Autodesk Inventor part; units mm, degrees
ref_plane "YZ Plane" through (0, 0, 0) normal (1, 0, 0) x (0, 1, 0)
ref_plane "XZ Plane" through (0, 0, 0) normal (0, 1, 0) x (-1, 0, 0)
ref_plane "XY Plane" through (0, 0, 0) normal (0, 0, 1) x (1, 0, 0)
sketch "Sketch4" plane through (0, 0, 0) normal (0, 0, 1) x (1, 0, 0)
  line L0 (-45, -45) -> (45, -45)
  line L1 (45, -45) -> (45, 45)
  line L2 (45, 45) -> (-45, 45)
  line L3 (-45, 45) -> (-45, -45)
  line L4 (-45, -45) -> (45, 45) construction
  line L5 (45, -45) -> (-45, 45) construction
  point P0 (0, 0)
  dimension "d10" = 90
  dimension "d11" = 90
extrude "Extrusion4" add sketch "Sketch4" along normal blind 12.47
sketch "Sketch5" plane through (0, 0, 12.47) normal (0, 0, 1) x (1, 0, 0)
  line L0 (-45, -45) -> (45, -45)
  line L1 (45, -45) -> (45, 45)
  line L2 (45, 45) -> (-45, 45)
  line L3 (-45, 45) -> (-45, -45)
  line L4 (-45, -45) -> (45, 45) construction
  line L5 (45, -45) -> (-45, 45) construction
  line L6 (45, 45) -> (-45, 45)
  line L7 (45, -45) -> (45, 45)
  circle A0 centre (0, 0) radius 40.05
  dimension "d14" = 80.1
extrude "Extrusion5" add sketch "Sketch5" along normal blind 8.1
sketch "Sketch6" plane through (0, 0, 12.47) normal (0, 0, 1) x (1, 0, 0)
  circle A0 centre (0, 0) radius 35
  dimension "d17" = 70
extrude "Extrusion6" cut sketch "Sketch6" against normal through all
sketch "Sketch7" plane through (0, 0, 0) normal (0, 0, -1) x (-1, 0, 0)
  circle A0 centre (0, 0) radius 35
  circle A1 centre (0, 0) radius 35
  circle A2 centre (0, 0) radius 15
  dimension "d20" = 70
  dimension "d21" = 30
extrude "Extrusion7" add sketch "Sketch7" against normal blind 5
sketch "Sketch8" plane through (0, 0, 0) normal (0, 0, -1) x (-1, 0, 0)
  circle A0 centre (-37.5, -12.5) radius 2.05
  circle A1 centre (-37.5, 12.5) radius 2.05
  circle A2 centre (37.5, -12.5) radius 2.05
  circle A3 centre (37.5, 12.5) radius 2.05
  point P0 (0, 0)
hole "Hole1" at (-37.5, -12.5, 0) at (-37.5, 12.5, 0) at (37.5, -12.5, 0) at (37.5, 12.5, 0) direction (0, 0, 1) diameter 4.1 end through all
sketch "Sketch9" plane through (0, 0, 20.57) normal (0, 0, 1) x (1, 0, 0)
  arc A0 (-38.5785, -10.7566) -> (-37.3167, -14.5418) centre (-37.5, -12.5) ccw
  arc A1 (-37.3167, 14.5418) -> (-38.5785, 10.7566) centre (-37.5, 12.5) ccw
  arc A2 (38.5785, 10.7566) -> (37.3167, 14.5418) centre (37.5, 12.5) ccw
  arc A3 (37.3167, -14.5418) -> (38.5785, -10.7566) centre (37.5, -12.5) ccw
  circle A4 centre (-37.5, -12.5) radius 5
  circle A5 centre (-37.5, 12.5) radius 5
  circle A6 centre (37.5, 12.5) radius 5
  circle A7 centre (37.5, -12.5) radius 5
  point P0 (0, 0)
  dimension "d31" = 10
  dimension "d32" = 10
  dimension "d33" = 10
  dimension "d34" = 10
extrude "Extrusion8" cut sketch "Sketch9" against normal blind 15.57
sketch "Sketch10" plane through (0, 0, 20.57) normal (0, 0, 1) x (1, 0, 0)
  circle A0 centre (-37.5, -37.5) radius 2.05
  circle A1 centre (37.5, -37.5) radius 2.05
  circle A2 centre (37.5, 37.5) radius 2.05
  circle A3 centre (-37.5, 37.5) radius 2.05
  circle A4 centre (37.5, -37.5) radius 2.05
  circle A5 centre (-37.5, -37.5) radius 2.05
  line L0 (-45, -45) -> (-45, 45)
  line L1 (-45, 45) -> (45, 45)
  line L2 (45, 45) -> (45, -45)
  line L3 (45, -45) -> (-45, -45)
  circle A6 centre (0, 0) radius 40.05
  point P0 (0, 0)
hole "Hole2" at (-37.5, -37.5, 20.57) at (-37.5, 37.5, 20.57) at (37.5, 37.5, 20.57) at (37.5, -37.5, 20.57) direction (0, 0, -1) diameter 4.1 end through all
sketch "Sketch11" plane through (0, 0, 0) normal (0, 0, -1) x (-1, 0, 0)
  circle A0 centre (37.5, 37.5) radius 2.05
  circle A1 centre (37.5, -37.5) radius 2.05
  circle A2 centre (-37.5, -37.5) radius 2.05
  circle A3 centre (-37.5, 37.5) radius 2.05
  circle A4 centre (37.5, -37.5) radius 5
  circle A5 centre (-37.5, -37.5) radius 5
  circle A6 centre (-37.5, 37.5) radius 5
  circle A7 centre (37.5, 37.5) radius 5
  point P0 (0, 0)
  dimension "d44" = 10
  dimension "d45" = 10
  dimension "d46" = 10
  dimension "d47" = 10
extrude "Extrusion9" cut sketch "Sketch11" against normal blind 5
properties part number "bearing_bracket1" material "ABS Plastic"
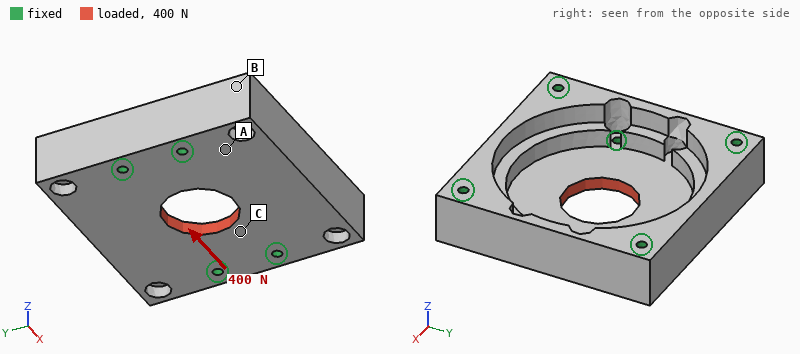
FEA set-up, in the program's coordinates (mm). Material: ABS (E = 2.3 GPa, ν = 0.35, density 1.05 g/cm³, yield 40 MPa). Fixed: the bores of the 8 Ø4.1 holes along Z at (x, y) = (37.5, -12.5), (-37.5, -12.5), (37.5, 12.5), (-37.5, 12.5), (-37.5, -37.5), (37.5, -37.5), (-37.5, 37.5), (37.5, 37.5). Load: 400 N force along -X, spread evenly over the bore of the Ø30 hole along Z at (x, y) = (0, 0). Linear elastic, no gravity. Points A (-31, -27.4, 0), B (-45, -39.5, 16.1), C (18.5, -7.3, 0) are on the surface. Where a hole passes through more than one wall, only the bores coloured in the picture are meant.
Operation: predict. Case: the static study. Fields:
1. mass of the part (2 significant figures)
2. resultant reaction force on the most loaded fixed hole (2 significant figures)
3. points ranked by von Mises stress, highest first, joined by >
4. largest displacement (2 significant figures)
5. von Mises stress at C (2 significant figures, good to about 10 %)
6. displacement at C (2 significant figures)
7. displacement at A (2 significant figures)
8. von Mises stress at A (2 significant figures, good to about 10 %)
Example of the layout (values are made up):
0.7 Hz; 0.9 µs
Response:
92 g; 66 N; C > A > B; 11 µm; 0.80 MPa; 8.0 µm; 2.8 µm; 0.29 MPa
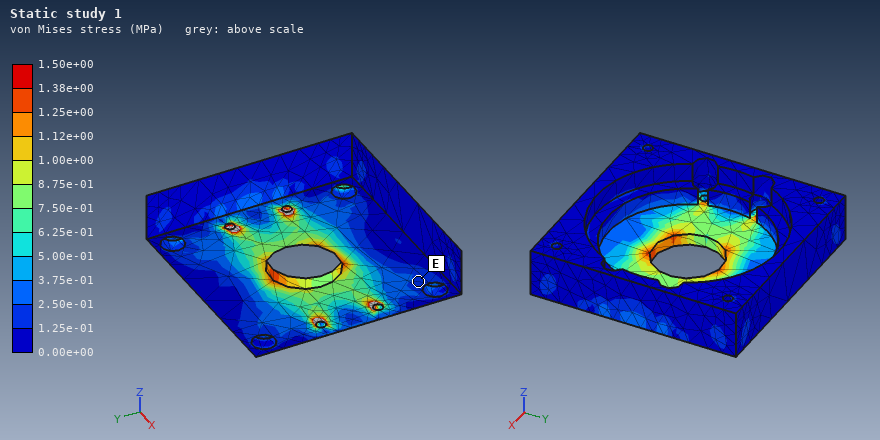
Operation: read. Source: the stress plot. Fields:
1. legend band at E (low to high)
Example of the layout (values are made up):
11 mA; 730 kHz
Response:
1.25e-01 to 2.50e-01 MPa
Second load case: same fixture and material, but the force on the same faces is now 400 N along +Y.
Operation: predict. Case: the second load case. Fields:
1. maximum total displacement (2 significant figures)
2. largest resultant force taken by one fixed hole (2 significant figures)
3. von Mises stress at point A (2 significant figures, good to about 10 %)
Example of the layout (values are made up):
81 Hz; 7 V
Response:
22 µm; 58 N; 0.58 MPa
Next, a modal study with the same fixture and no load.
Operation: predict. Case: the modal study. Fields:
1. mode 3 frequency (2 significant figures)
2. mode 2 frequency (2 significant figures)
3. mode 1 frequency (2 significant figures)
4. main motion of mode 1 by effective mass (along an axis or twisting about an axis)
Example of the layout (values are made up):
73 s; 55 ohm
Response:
3800 Hz; 3300 Hz; 2800 Hz; along Z
